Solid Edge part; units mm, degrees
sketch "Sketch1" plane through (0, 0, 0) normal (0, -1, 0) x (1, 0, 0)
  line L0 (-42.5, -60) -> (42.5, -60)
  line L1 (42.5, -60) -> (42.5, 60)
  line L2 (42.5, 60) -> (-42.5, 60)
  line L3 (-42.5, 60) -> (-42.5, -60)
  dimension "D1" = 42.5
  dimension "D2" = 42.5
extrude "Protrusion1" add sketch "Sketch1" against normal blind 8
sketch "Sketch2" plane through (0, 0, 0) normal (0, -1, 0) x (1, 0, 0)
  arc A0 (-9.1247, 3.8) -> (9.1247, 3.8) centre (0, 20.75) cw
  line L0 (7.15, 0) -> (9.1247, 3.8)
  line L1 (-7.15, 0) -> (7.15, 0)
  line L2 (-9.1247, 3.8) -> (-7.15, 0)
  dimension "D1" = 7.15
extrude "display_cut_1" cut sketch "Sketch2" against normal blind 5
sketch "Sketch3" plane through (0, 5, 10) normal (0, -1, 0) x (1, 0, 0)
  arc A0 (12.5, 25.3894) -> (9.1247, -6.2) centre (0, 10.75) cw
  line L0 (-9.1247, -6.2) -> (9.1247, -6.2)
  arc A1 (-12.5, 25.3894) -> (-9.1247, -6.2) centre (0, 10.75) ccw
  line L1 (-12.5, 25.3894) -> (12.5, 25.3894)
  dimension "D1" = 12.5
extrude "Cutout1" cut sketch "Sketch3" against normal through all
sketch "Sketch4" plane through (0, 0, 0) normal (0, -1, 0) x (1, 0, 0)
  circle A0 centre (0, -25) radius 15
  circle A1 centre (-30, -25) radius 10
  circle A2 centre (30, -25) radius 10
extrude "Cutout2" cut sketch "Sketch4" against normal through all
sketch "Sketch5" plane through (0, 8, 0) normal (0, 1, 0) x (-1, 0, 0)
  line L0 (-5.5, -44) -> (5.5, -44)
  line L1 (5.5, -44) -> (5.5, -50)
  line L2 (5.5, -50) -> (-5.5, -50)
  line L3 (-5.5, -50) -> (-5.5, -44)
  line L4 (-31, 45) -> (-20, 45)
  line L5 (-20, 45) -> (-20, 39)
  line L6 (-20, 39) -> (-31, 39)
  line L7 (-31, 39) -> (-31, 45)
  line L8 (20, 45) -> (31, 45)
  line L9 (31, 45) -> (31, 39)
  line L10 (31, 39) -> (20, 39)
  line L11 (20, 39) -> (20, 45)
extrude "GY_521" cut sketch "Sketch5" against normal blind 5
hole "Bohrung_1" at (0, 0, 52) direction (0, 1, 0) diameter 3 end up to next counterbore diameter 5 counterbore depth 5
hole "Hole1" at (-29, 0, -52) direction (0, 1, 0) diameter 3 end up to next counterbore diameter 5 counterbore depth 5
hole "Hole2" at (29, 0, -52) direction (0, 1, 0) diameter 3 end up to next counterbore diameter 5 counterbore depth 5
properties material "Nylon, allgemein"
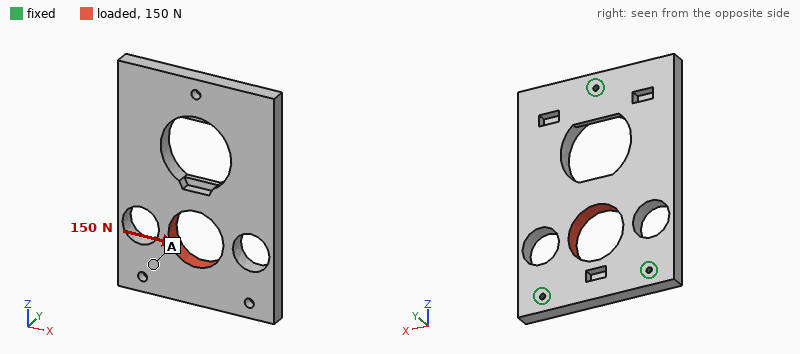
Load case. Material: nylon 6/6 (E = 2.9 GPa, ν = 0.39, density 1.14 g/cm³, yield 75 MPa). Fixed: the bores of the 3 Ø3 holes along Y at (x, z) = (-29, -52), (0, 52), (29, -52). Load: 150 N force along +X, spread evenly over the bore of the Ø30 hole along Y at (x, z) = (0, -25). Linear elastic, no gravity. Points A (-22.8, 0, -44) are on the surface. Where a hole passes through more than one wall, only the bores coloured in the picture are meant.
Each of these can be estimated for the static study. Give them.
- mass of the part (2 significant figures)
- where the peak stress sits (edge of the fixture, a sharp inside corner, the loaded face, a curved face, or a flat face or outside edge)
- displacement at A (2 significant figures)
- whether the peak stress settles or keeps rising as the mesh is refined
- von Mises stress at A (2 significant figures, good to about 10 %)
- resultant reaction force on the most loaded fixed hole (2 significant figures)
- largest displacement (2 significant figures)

69 g
edge of the fixture
5.8 µm
keeps rising
0.30 MPa
59 N
26 µm
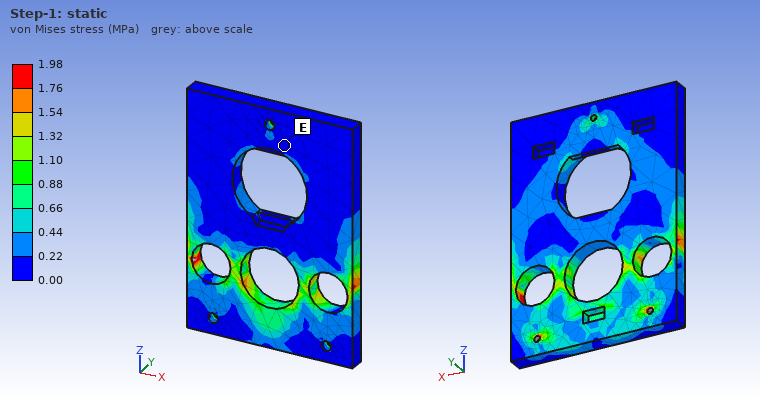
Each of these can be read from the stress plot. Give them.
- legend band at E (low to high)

0.00 to 0.22 MPa
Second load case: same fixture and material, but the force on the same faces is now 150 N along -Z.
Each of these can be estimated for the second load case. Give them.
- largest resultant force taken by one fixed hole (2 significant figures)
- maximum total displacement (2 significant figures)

59 N
22 µm
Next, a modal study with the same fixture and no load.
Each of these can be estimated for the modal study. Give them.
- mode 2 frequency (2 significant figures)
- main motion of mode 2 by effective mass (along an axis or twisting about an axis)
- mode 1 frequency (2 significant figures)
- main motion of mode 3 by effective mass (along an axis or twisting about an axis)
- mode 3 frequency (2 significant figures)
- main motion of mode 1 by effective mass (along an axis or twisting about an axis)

590 Hz
along Y
440 Hz
twisting about X
1200 Hz
twisting about Z
